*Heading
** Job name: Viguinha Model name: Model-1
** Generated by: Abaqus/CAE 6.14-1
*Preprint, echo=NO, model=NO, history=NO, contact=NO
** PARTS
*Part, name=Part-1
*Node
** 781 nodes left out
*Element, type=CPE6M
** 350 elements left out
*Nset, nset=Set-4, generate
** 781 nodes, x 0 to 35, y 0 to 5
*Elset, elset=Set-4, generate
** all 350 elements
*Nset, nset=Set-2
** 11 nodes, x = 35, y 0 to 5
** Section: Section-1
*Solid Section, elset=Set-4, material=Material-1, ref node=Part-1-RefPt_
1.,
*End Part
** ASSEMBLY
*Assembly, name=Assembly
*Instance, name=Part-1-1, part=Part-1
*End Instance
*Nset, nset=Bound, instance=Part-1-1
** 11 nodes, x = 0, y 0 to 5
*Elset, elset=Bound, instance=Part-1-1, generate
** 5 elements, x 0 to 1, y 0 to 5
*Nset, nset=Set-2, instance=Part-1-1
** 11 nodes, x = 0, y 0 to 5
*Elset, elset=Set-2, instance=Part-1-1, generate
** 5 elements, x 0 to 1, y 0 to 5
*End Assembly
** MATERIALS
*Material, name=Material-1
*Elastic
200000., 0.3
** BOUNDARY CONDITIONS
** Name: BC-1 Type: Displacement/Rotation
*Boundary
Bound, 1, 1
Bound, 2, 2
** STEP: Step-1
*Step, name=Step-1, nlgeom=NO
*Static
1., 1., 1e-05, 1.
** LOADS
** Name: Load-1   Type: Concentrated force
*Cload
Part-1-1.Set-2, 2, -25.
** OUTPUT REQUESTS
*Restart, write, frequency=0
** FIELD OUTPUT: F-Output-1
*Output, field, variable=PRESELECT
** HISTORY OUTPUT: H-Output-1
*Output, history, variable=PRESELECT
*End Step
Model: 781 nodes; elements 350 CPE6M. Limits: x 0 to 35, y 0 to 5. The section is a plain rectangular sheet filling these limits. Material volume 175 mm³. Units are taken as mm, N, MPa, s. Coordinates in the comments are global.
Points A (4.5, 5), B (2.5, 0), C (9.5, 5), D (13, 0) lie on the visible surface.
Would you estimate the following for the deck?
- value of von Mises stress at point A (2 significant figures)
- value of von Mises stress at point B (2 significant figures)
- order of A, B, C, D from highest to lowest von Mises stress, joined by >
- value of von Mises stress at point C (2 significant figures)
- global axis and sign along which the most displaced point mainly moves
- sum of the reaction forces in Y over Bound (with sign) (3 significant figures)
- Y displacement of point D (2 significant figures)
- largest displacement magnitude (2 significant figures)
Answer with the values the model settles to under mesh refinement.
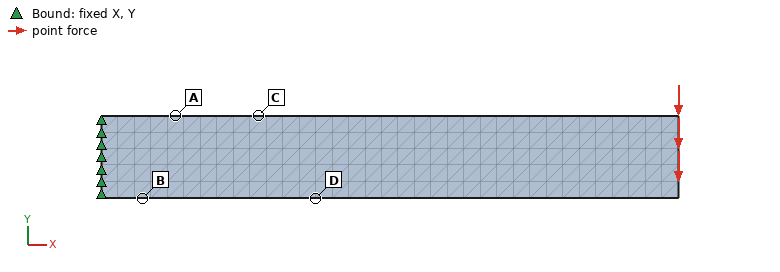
1800 MPa
1900 MPa
B > A > C > D
1500 MPa
-Y
275 N
-0.32 mm
1.7 mm
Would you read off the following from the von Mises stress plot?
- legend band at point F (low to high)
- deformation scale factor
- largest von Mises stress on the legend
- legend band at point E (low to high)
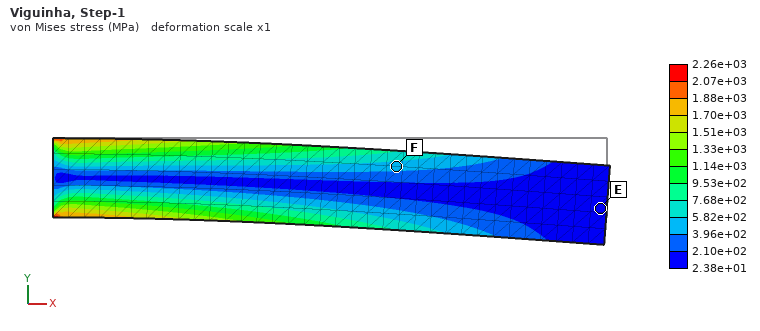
3.96e+02 to 5.82e+02 MPa
1
2.26e+03 MPa
2.38e+01 to 2.10e+02 MPa
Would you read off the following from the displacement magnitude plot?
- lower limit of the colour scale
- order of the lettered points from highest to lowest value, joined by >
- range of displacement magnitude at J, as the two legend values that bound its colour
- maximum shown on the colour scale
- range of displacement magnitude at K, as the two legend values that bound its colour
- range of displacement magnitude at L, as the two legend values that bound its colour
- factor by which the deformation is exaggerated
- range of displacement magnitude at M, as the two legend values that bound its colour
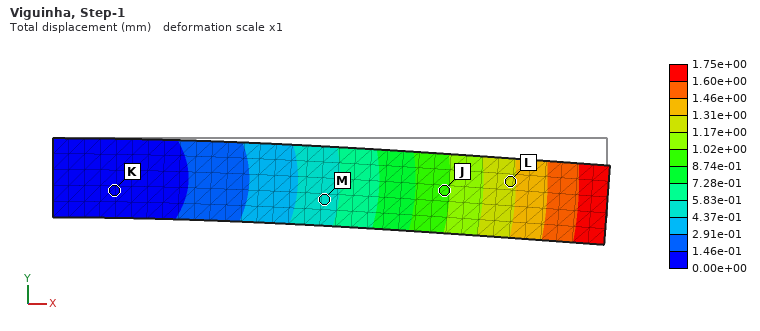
0.00e+00 mm
L > J > M > K
8.74e-01 to 1.02e+00 mm
1.75e+00 mm
0.00e+00 to 1.46e-01 mm
1.17e+00 to 1.31e+00 mm
1
4.37e-01 to 5.83e-01 mm
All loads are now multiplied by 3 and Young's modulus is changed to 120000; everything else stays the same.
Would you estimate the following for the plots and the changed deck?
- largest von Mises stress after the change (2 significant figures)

6800 MPa
